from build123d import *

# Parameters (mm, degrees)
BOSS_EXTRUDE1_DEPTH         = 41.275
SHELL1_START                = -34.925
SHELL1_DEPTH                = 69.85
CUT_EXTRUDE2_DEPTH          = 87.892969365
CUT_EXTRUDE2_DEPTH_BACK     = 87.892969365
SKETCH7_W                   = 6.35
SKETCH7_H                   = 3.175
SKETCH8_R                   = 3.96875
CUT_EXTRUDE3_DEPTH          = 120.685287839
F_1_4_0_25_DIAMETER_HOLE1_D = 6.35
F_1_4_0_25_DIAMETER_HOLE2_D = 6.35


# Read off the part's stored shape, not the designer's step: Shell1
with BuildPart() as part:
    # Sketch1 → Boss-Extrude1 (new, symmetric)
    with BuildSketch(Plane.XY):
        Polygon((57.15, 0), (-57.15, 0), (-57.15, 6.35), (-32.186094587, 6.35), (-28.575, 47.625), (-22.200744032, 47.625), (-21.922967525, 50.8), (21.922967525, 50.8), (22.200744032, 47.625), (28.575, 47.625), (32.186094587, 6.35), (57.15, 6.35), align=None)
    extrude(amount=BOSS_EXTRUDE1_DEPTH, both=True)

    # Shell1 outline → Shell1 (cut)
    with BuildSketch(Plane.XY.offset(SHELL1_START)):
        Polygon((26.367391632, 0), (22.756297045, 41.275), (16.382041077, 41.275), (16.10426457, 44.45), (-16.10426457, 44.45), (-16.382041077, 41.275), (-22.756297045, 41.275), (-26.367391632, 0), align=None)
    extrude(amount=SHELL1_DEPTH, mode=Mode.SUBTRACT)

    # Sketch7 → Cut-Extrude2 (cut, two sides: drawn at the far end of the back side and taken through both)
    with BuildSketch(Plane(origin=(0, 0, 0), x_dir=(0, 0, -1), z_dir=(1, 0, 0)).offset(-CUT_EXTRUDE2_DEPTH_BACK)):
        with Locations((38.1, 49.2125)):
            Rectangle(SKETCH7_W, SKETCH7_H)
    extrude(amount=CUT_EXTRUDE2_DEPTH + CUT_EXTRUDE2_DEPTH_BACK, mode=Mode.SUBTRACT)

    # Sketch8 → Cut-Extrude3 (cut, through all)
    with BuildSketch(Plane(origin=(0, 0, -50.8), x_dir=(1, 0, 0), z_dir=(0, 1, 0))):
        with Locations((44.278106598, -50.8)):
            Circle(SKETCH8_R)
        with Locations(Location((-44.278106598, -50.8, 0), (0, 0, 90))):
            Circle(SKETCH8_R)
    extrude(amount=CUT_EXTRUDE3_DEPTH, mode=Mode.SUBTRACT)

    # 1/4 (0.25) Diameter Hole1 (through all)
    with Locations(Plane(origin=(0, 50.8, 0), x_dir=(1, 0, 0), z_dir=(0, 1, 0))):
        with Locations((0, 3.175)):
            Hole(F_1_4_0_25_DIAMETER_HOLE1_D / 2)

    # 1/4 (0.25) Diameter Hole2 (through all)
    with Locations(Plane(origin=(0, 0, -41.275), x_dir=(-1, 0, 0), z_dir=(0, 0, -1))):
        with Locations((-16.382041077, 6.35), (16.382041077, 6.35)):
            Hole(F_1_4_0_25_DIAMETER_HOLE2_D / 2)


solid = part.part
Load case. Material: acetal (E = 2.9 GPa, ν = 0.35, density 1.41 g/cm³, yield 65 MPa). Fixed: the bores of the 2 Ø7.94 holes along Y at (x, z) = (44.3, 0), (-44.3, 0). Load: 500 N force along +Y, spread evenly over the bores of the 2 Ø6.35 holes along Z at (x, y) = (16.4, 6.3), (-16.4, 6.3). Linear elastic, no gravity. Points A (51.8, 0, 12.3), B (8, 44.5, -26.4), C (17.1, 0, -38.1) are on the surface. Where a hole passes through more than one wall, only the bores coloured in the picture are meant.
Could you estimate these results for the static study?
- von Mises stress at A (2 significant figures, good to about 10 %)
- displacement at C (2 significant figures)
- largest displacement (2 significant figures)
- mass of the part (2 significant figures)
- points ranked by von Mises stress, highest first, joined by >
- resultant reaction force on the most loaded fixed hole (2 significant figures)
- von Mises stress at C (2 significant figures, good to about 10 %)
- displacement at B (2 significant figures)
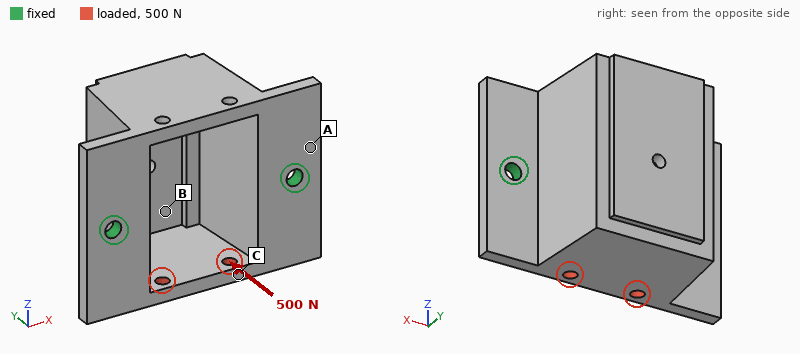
9.4 MPa
0.98 mm
1.5 mm
180 g
A > C > B
270 N
6.5 MPa
1.2 mm
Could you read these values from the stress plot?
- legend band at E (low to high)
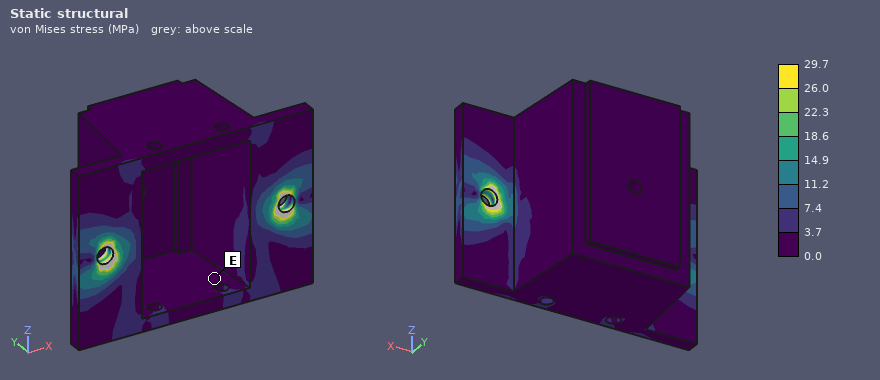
0.0 to 3.7 MPa
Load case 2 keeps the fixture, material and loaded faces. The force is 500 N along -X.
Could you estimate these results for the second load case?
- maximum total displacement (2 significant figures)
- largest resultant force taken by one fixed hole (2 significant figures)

0.28 mm
270 N
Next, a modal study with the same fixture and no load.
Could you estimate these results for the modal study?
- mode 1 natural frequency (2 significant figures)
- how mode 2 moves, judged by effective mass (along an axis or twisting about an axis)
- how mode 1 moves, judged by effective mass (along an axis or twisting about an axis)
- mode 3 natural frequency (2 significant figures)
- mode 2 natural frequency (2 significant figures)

280 Hz
along X
along Z
1000 Hz
970 Hz
